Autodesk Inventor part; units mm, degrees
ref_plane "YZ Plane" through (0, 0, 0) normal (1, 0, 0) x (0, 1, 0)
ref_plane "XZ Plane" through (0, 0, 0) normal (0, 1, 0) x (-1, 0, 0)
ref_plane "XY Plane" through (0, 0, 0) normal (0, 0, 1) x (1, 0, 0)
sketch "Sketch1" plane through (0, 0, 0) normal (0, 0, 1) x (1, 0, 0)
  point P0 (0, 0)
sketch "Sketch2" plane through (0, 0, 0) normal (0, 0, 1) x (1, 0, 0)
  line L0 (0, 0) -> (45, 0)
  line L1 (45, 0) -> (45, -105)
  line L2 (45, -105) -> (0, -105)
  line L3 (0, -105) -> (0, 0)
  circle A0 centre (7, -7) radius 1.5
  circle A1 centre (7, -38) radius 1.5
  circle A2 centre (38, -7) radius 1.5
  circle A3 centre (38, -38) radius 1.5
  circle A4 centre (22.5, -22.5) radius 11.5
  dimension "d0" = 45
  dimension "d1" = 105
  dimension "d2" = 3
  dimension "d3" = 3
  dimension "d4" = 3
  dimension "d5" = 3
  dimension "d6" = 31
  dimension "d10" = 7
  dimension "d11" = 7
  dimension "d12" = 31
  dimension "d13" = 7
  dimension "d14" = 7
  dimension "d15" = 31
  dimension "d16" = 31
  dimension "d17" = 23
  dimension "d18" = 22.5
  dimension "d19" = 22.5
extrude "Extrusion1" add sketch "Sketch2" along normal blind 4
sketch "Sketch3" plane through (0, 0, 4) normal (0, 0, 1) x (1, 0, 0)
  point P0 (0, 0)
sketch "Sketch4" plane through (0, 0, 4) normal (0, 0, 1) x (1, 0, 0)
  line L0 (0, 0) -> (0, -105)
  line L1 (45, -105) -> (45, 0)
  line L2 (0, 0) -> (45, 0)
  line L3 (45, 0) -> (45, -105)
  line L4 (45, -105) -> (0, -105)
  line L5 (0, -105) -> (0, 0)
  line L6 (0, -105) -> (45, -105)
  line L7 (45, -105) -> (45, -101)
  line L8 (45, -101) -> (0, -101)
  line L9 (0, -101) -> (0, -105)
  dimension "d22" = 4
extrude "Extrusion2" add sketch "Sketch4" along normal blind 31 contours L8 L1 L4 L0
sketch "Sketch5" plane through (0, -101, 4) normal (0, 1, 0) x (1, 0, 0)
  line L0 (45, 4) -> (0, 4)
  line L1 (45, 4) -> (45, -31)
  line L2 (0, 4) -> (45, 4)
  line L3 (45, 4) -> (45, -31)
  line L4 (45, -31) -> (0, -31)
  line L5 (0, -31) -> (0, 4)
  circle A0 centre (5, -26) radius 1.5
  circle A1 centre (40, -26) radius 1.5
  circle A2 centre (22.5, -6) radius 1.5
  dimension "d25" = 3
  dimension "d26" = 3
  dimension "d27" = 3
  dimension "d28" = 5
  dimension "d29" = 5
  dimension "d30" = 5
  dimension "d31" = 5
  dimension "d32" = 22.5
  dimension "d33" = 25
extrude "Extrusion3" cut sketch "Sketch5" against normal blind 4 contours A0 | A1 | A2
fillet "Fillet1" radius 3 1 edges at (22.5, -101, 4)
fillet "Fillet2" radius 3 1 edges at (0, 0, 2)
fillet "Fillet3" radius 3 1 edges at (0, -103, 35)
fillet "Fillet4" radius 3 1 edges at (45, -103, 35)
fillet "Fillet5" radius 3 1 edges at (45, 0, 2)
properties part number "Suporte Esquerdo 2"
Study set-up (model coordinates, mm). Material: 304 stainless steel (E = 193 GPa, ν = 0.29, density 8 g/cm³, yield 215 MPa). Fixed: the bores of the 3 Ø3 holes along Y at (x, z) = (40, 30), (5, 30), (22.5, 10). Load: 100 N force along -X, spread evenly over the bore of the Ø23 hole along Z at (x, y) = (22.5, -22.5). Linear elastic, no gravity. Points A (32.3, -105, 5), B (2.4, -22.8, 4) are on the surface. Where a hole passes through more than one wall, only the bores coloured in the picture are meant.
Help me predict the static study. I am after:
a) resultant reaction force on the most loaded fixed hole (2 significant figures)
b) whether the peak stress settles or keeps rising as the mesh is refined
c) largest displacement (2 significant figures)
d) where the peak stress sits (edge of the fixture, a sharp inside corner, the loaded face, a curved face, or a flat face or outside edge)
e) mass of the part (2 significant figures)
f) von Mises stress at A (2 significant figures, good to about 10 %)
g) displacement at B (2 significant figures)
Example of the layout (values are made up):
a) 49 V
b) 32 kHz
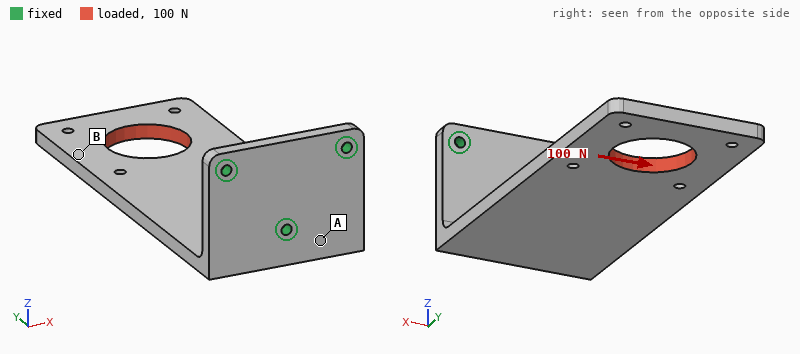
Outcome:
a) 110 N
b) keeps rising
c) 0.10 mm
d) edge of the fixture
e) 180 g
f) 18 MPa
g) 0.082 mm
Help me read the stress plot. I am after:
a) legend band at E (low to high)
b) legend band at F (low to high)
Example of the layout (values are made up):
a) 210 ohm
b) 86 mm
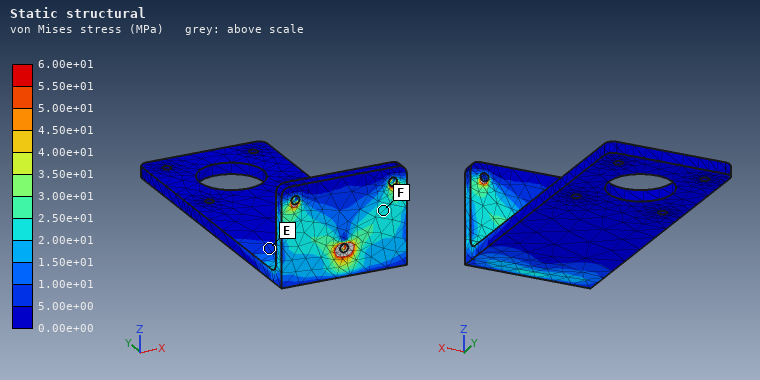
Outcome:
a) 5.00e+00 to 1.00e+01 MPa
b) 2.00e+01 to 2.50e+01 MPa
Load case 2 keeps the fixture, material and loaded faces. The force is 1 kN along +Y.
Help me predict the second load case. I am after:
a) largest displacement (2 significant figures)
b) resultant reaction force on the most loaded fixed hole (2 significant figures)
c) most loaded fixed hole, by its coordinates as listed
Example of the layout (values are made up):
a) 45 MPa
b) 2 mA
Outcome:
a) 0.12 mm
b) 1.2 kN
c) (22.5, 10)
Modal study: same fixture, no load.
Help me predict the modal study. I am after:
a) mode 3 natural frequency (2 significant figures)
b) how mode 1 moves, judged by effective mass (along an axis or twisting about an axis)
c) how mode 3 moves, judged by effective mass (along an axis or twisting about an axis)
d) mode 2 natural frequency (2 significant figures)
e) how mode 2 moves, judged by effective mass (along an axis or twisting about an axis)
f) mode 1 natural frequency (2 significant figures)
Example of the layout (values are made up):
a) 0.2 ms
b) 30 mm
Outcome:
a) 1400 Hz
b) along Z
c) twisting about Y
d) 670 Hz
e) along X
f) 300 Hz
